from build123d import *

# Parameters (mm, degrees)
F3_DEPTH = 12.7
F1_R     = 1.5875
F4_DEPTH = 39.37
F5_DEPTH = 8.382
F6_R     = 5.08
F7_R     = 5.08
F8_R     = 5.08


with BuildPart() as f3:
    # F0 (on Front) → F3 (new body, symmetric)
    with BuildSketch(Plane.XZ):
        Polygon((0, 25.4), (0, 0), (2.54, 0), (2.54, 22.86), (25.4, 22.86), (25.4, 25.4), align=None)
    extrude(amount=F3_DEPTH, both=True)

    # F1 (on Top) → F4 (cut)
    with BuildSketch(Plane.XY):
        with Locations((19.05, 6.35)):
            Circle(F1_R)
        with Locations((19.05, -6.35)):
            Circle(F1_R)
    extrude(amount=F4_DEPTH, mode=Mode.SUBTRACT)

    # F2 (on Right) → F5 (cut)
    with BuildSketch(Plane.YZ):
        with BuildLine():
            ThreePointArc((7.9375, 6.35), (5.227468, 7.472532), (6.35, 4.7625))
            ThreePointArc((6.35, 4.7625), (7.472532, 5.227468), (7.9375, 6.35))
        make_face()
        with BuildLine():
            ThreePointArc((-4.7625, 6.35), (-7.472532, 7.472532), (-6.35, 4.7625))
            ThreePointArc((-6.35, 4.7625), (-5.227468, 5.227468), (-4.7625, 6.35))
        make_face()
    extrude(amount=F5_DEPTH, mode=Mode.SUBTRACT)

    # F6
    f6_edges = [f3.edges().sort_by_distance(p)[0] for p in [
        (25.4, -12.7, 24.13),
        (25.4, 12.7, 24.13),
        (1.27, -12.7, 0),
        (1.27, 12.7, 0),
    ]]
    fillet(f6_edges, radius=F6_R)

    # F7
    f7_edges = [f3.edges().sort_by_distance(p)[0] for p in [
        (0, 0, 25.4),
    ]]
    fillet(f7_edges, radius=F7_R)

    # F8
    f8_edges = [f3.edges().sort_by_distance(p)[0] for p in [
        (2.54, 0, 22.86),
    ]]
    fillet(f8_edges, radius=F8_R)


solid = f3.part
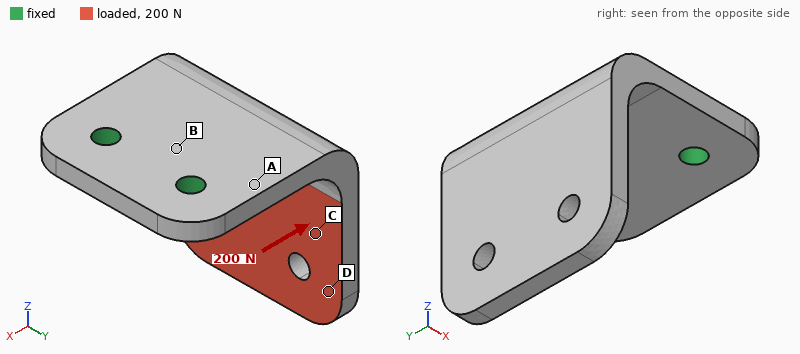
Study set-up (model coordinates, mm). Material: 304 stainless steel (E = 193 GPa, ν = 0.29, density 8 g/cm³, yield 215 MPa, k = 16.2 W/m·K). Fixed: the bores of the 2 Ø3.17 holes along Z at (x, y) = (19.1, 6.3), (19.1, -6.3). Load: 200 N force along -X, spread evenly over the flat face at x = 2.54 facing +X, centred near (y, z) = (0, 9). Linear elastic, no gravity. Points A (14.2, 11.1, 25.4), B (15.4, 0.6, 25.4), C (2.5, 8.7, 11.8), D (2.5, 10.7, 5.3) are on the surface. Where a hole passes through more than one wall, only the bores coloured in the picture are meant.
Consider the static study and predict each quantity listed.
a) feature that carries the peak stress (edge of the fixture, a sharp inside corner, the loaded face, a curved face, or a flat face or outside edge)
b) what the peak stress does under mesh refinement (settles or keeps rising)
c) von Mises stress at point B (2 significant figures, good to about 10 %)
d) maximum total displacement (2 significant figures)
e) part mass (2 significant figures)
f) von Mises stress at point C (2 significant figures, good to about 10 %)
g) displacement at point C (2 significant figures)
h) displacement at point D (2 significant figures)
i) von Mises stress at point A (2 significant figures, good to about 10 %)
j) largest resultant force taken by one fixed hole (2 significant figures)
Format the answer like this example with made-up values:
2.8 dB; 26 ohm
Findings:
edge of the fixture; keeps rising; 85 MPa; 0.20 mm; 24 g; 26 MPa; 0.10 mm; 0.15 mm; 100 MPa; 100 N
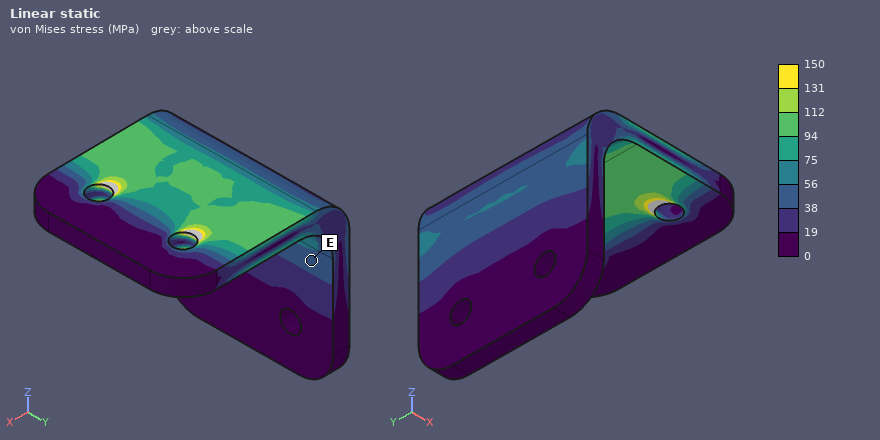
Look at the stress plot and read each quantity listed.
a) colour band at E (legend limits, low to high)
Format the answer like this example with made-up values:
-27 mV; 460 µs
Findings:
38 to 56 MPa
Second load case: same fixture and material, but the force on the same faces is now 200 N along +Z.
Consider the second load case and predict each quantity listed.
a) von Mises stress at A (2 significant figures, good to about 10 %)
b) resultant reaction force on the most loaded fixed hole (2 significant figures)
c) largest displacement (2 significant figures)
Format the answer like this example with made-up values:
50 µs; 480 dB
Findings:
79 MPa; 100 N; 96 µm
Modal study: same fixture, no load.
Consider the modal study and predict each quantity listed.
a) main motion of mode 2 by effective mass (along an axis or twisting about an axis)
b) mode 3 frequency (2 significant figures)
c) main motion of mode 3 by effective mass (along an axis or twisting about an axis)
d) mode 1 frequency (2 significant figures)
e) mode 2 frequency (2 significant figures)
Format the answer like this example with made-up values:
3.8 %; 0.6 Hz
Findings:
along Y; 5600 Hz; along Z; 1800 Hz; 3300 Hz
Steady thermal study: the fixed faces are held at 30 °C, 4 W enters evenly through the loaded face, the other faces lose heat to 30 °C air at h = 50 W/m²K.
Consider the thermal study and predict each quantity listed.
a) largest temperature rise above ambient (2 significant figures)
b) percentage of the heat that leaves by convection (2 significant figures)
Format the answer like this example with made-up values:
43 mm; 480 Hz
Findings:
55 K; 64 %
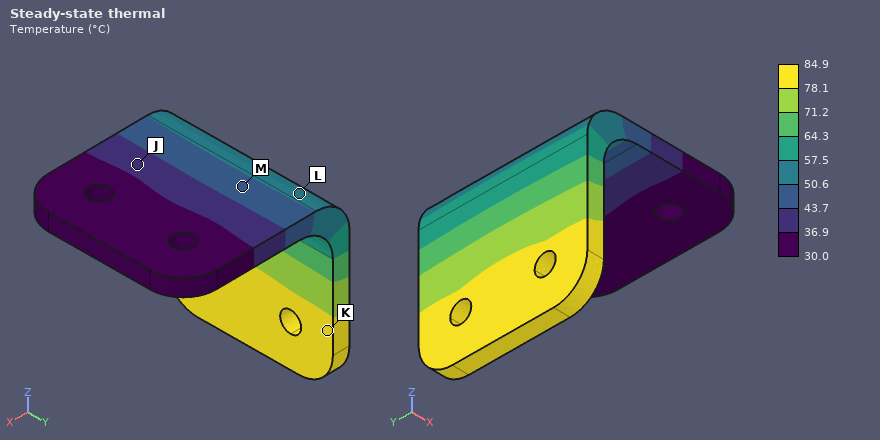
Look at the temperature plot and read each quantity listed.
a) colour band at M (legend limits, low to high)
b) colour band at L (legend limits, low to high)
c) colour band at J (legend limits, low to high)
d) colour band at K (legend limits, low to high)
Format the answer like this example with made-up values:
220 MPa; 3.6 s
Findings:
43.7 to 50.6 °C; 50.6 to 57.5 °C; 36.9 to 43.7 °C; 78.1 to 84.9 °C
